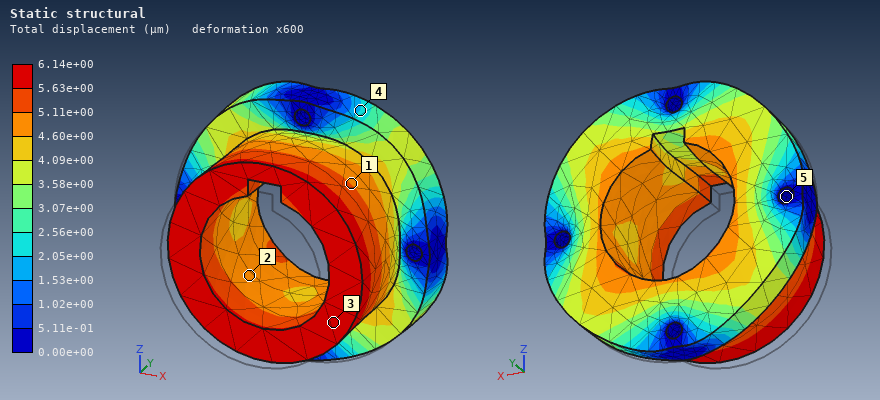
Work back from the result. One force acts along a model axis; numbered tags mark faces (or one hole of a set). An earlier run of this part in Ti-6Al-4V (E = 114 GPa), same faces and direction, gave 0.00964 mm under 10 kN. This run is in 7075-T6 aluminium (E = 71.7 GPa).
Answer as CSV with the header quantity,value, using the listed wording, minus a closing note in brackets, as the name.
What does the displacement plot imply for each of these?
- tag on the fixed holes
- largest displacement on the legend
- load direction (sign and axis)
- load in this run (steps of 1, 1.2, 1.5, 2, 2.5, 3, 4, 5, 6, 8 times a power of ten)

quantity,value
tag on the fixed holes,5
largest displacement on the legend,6.14e+00 µm
load direction,+Y
load in this run,4 kN
